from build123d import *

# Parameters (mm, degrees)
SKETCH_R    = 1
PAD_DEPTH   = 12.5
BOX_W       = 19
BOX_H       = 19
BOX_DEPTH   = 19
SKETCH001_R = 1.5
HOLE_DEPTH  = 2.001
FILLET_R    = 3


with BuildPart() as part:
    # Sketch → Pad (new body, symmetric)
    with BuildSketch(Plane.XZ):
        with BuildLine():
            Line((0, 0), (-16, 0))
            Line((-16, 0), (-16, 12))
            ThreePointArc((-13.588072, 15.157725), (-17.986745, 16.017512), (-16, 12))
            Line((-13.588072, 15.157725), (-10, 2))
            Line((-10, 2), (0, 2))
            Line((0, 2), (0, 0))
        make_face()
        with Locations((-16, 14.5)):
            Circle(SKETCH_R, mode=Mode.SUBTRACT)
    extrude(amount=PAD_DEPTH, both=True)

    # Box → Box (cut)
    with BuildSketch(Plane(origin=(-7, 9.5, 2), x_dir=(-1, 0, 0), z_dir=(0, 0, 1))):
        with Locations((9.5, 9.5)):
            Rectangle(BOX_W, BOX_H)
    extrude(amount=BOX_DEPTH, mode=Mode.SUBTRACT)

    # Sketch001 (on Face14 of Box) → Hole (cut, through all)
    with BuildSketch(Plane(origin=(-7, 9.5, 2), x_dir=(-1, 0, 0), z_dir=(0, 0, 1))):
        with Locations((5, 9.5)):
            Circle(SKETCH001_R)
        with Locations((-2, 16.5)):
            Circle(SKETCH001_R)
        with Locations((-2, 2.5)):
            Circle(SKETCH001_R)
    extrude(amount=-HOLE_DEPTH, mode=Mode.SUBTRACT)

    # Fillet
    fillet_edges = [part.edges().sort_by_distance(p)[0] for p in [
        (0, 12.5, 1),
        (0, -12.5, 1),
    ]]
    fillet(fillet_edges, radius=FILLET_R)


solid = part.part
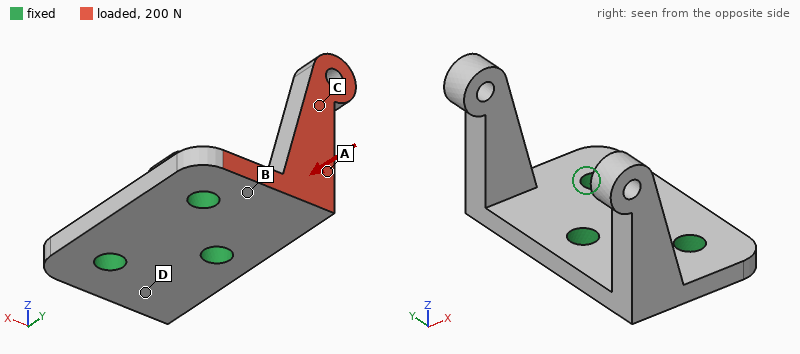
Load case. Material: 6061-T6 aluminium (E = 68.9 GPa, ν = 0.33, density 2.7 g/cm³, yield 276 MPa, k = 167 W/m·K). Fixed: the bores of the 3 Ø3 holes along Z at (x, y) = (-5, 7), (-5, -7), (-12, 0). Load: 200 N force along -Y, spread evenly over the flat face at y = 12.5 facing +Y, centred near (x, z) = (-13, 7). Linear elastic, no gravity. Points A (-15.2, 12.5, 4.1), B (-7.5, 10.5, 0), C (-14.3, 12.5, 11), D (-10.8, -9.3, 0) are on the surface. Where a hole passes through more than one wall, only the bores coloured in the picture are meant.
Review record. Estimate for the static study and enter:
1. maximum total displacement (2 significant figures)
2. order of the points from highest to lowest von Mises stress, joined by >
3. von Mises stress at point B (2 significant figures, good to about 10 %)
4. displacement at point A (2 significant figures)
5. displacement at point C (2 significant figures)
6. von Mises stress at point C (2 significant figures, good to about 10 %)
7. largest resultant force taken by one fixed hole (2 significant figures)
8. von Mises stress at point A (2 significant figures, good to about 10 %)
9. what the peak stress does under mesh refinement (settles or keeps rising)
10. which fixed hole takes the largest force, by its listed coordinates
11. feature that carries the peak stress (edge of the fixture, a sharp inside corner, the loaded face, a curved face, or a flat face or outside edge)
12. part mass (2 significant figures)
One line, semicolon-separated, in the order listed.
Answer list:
0.28 mm; B > A > C > D; 120 MPa; 0.082 mm; 0.17 mm; 31 MPa; 170 N; 81 MPa; keeps rising; (-12, 0); edge of the fixture; 3.1 g
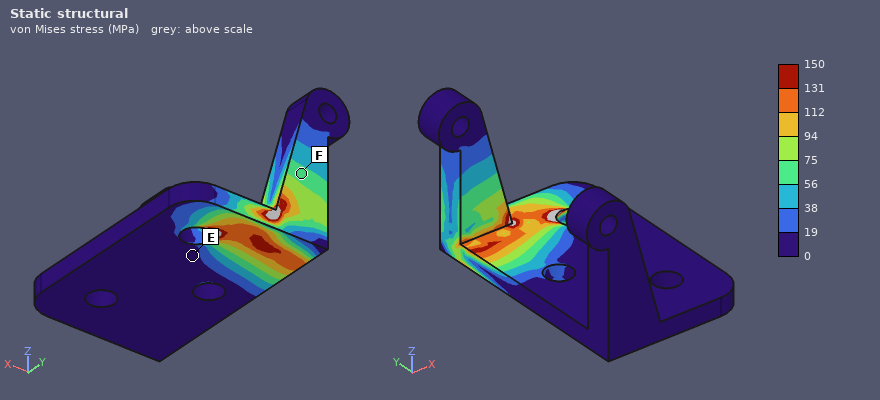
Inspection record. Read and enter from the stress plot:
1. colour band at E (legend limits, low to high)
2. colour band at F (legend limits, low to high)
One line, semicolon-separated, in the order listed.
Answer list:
0 to 19 MPa; 56 to 75 MPa
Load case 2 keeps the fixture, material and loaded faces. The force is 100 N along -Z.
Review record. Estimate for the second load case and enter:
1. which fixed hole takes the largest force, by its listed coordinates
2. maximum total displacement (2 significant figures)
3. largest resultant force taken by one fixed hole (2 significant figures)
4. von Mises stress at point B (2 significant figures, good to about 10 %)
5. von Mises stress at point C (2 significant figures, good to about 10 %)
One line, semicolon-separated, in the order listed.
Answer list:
(-5, 7); 0.13 mm; 80 N; 64 MPa; 9.1 MPa
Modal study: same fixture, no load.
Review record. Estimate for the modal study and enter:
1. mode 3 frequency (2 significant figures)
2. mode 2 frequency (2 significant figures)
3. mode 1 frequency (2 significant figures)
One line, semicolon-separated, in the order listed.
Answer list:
8100 Hz; 5500 Hz; 5400 Hz
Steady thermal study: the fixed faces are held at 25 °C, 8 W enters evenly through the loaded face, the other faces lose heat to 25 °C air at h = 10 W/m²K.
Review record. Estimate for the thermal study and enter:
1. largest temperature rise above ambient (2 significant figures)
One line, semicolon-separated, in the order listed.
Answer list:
34 K
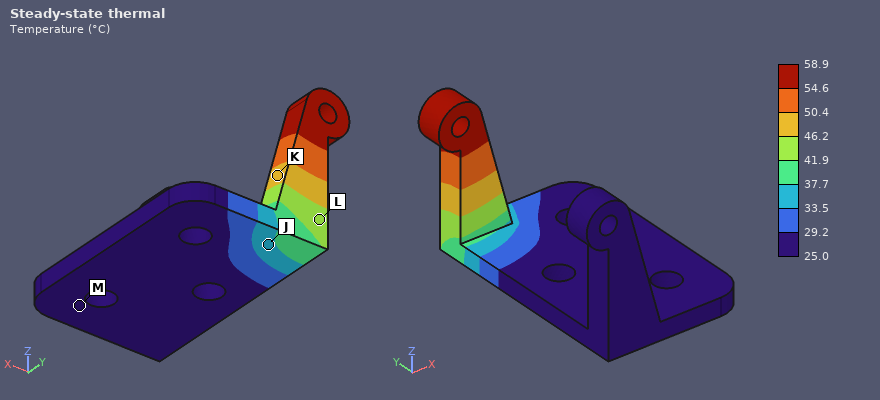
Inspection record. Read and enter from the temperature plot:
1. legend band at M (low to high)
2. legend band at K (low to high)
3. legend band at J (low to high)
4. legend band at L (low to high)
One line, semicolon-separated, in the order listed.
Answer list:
25.0 to 29.2 °C; 46.2 to 50.4 °C; 33.5 to 37.7 °C; 41.9 to 46.2 °C
